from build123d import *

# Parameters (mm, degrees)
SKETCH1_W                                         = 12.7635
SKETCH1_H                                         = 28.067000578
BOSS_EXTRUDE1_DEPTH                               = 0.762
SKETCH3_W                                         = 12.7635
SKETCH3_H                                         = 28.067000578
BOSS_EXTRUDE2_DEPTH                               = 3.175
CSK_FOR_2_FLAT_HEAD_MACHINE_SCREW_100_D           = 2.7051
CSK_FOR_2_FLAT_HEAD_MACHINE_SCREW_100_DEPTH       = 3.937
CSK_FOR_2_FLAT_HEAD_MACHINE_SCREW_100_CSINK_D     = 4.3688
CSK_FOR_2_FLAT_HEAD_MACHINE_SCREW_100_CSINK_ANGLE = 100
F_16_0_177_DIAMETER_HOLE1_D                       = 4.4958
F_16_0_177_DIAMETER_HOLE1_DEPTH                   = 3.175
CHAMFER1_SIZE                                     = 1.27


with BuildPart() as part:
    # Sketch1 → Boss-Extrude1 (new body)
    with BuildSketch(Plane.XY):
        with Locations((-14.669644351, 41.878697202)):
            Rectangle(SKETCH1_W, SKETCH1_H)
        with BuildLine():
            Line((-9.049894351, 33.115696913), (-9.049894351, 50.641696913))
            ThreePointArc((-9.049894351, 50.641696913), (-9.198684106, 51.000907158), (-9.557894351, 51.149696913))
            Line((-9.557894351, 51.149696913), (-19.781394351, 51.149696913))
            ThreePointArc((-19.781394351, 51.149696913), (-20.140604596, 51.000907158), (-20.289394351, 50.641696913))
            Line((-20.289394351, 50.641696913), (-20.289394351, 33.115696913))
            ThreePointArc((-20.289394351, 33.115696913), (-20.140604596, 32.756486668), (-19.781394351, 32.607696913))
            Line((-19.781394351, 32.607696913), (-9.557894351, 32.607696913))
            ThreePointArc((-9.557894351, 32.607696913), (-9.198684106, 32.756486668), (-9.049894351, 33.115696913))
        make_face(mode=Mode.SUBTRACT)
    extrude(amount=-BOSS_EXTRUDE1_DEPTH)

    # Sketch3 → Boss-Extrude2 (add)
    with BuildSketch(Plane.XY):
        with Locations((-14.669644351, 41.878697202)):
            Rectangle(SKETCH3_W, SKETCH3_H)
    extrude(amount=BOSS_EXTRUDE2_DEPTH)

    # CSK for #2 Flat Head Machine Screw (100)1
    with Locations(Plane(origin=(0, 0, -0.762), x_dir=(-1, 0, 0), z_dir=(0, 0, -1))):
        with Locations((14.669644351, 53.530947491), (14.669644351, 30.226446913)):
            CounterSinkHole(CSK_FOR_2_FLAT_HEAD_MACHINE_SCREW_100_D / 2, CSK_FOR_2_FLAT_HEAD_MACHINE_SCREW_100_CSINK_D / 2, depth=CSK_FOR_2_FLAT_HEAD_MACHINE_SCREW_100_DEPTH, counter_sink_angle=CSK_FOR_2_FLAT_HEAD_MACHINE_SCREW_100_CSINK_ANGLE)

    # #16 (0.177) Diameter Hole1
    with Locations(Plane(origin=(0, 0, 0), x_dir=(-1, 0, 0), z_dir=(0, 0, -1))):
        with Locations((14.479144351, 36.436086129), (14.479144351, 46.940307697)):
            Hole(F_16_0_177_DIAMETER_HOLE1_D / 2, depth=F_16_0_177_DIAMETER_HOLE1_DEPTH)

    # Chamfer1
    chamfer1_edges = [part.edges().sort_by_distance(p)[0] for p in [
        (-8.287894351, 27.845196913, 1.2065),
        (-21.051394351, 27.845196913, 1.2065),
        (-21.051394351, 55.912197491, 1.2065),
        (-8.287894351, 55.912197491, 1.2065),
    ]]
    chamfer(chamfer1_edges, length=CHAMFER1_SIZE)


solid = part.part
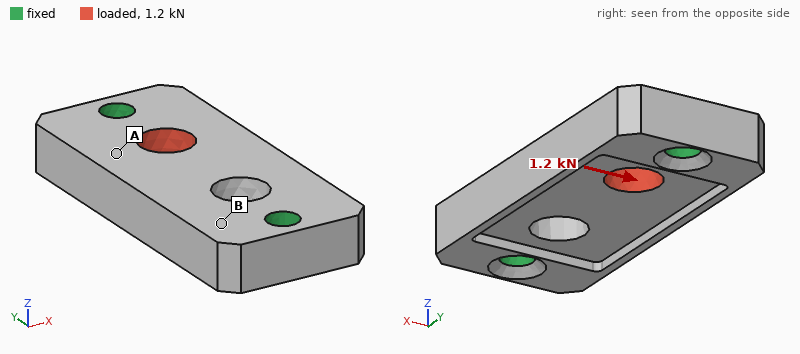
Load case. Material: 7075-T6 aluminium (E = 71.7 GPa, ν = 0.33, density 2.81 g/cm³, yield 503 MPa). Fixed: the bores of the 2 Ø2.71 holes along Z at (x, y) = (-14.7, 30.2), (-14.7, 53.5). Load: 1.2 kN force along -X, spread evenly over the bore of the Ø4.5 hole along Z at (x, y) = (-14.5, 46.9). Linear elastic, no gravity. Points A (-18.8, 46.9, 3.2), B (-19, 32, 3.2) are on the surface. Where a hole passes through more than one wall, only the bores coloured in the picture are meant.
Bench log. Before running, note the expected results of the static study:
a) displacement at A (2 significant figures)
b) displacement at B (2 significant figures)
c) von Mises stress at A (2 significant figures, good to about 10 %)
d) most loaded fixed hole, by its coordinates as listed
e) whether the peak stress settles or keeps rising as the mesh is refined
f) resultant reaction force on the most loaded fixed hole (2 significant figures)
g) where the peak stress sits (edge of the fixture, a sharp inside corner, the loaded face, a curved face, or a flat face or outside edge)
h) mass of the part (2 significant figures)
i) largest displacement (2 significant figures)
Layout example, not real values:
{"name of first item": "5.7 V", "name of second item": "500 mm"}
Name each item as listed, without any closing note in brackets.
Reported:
{"displacement at A": "9.0 µm", "displacement at B": "2.0 µm", "von Mises stress at A": "39 MPa", "most loaded fixed hole, by its coordinates as listed": "(-14.7, 53.5)", "whether the peak stress settles or keeps rising as the mesh is refined": "keeps rising", "resultant reaction force on the most loaded fixed hole": "890 N", "where the peak stress sits": "edge of the fixture", "mass of the part": "3.1 g", "largest displacement": "11 µm"}
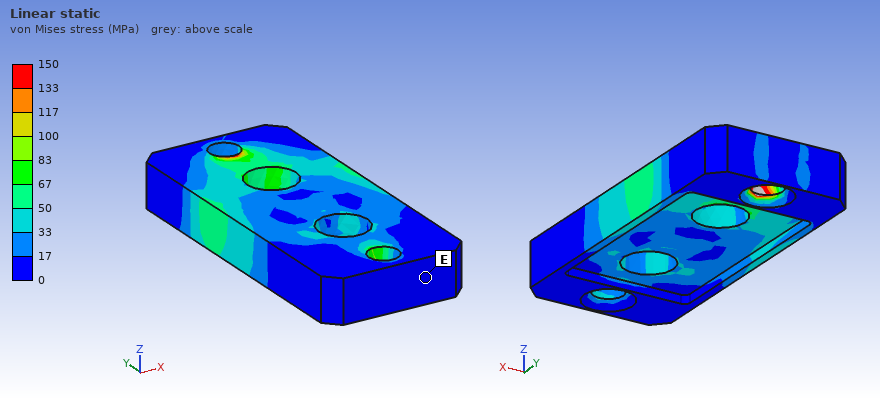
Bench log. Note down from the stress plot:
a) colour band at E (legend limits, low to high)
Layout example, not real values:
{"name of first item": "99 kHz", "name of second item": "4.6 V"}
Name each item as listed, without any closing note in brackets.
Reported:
{"colour band at E": "0 to 17 MPa"}
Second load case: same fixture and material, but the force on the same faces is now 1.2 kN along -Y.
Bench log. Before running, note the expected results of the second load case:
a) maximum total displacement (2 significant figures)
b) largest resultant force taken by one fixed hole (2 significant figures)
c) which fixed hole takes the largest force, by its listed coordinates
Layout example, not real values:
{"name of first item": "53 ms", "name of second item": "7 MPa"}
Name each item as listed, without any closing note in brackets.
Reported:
{"maximum total displacement": "5.0 µm", "largest resultant force taken by one fixed hole": "830 N", "which fixed hole takes the largest force, by its listed coordinates": "(-14.7, 53.5)"}
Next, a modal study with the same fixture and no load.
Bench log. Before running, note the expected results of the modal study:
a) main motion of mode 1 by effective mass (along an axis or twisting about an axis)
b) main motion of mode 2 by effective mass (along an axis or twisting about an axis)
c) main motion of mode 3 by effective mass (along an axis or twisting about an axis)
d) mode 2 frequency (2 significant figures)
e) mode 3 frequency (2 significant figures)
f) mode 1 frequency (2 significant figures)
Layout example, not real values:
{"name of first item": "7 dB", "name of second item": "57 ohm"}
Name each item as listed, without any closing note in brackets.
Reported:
{"main motion of mode 1 by effective mass": "along Z", "main motion of mode 2 by effective mass": "twisting about Y", "main motion of mode 3 by effective mass": "along X", "mode 2 frequency": "30 kHz", "mode 3 frequency": "42 kHz", "mode 1 frequency": "26 kHz"}
